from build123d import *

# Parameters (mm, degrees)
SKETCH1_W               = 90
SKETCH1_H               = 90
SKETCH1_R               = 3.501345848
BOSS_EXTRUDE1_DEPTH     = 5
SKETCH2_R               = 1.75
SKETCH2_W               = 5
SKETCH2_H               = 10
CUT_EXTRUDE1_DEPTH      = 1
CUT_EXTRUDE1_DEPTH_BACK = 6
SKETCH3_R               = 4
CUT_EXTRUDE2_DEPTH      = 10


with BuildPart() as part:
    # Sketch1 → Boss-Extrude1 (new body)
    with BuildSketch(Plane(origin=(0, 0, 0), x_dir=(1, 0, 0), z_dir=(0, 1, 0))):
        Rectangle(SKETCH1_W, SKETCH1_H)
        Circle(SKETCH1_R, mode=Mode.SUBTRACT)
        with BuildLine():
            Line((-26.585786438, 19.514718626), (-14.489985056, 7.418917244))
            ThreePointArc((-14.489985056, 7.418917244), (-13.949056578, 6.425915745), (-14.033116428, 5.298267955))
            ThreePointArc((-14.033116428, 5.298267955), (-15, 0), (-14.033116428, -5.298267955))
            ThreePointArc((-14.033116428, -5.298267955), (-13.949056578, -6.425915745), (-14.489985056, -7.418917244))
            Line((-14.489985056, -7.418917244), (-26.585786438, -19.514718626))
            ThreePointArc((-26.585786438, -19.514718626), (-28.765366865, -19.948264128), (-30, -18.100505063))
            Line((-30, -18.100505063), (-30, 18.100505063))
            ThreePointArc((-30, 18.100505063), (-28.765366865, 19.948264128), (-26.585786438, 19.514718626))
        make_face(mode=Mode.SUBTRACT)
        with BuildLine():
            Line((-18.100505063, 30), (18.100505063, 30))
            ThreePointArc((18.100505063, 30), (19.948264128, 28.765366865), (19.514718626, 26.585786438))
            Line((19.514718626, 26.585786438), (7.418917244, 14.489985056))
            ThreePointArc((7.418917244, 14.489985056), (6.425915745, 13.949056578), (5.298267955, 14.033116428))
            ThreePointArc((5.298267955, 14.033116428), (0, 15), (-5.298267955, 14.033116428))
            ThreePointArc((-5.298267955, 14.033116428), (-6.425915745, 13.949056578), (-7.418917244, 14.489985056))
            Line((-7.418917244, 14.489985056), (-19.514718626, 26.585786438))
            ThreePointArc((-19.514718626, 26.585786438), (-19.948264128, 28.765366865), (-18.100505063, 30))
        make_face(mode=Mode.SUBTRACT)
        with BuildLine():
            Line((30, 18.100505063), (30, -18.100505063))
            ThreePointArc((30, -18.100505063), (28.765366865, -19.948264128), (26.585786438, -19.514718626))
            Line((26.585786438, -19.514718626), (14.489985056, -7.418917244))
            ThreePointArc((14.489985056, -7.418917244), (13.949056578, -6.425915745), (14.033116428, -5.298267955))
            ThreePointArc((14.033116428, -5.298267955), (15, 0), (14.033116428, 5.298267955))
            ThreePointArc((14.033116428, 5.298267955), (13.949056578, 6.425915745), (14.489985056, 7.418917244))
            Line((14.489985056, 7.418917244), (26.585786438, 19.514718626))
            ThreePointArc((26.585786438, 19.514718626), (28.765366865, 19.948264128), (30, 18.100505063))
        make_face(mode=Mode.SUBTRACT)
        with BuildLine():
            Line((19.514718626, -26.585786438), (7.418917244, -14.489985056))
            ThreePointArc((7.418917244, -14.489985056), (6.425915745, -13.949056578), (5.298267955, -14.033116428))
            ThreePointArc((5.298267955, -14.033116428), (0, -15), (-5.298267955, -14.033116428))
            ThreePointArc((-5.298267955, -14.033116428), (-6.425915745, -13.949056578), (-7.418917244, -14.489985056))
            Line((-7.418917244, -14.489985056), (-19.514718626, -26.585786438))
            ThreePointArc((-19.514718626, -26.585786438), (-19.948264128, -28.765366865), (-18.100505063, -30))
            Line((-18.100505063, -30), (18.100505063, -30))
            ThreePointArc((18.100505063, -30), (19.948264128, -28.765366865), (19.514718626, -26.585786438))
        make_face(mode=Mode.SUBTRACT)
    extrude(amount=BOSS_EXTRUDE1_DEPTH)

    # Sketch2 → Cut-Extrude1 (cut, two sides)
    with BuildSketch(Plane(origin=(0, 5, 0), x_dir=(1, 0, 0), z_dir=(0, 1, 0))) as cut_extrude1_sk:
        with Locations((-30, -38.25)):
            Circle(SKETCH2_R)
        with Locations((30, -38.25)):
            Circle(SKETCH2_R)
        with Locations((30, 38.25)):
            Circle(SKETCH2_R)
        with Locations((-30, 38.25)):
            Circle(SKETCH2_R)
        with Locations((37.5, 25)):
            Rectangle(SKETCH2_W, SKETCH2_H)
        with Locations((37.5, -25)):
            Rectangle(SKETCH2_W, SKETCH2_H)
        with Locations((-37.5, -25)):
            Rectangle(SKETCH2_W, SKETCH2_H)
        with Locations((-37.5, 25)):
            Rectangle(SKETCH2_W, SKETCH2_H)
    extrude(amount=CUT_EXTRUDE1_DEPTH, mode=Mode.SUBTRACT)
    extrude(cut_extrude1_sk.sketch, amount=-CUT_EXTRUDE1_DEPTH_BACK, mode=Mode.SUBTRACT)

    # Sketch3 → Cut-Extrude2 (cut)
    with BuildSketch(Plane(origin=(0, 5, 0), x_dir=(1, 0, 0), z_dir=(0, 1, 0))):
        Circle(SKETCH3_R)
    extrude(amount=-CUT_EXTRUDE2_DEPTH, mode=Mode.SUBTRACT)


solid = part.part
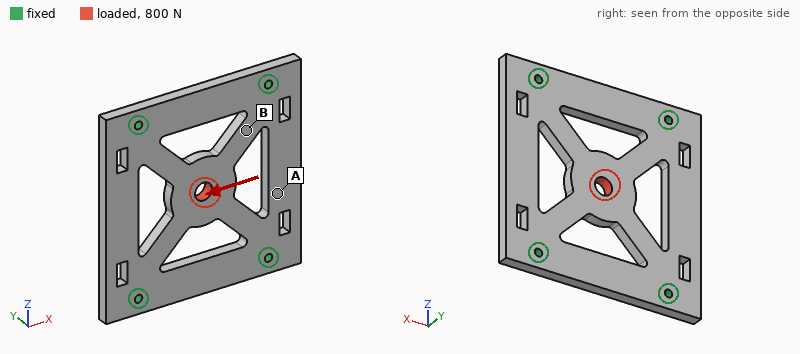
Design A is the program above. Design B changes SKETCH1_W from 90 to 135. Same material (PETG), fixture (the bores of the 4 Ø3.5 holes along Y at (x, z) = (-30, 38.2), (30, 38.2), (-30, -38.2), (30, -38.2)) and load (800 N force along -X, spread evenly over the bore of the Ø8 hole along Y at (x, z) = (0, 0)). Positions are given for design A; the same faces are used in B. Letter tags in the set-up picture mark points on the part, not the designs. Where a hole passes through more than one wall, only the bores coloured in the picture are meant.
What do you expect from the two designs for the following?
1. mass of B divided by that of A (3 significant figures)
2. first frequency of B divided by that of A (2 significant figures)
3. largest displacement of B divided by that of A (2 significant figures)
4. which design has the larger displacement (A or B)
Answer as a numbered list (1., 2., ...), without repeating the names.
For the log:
1. 1.68
2. 0.52
3. 0.92
4. A
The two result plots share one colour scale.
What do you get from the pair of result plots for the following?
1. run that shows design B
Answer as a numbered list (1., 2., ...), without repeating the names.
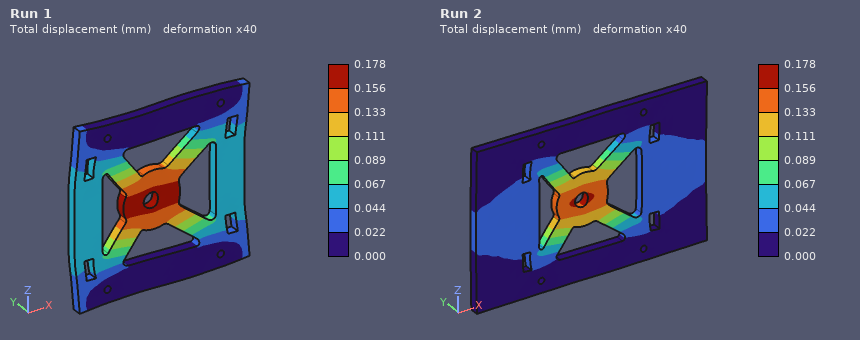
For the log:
1. Run 2
